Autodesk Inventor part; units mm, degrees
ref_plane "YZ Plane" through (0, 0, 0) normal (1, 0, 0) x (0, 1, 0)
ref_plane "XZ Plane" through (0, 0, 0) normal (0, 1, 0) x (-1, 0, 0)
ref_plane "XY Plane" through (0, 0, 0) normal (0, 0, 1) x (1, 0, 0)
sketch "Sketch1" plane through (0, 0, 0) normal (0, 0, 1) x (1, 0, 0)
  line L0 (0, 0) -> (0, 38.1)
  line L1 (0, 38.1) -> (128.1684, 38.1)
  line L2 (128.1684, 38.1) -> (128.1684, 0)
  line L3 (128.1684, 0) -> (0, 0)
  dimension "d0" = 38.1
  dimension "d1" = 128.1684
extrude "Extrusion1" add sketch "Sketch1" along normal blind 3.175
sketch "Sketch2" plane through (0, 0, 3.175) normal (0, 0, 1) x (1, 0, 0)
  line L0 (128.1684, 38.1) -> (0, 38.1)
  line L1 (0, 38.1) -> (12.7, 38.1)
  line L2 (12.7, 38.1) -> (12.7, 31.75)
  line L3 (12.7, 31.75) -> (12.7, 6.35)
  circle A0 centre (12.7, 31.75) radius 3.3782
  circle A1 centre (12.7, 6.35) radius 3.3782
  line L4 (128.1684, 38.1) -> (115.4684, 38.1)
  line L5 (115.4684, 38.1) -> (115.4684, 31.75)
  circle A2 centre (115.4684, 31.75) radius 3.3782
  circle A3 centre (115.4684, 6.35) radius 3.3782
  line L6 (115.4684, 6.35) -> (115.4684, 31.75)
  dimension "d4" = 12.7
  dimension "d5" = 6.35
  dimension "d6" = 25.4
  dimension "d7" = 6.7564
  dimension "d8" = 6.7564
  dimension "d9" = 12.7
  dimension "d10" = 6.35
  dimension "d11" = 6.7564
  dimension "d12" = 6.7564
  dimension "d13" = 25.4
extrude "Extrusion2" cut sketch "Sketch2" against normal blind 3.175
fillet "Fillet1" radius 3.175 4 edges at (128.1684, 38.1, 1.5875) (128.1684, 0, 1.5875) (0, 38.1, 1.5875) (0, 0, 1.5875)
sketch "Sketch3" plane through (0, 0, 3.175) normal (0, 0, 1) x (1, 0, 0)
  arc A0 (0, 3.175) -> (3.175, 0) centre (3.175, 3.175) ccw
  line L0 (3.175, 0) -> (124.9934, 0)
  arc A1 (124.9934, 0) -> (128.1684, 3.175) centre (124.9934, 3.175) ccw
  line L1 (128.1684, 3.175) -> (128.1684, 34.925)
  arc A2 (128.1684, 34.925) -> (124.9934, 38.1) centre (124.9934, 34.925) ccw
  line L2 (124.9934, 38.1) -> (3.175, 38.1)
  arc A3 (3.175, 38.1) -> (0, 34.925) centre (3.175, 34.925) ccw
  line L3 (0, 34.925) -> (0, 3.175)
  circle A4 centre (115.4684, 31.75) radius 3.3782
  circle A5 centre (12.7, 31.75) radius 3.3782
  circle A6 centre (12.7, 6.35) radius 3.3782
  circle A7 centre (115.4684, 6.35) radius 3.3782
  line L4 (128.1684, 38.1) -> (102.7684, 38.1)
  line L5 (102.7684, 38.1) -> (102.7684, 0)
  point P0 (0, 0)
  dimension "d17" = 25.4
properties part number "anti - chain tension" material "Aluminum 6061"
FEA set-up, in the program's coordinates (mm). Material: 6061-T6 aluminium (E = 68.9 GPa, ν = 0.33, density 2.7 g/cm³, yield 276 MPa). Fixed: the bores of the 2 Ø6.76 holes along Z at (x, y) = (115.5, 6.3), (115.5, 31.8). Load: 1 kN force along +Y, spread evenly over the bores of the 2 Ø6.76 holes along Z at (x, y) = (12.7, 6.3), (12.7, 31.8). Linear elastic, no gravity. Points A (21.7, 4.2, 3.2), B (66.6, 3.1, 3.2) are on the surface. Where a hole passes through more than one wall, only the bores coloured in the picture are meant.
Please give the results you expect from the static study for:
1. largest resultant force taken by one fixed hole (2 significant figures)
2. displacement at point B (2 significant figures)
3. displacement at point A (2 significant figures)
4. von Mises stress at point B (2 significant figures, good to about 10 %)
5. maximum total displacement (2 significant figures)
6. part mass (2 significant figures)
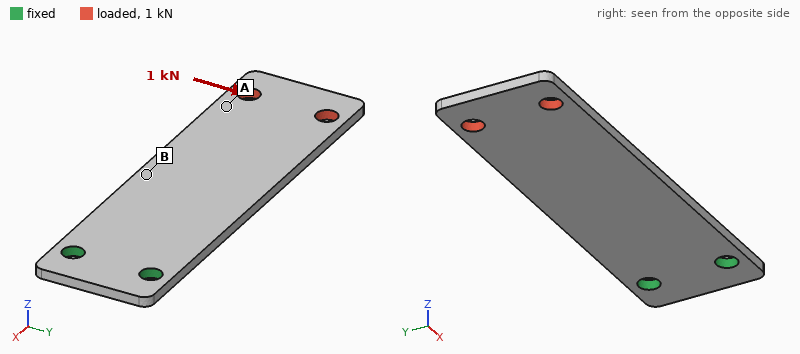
3.7 kN
0.13 mm
0.34 mm
59 MPa
0.46 mm
41 g
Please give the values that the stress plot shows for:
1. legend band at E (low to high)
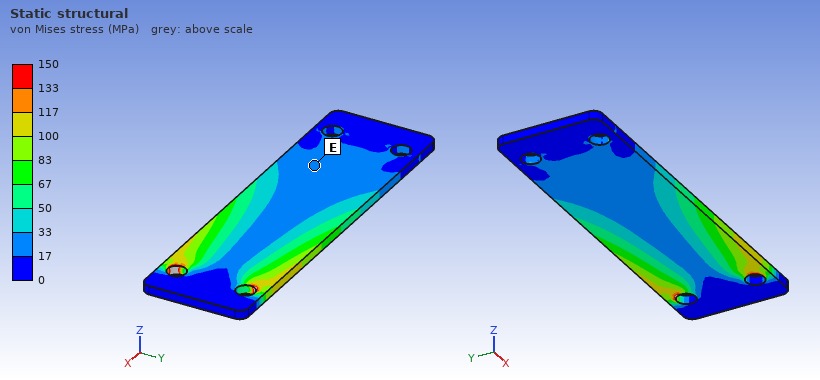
17 to 33 MPa
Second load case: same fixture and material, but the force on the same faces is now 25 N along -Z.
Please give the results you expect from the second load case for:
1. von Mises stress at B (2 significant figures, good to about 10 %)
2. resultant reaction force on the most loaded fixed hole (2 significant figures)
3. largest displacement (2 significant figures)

21 MPa
13 N
1.4 mm
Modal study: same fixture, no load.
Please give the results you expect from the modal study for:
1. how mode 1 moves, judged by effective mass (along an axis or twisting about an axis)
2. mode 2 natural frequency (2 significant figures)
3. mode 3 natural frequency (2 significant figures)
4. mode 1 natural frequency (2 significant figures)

along Z
1200 Hz
1300 Hz
210 Hz
